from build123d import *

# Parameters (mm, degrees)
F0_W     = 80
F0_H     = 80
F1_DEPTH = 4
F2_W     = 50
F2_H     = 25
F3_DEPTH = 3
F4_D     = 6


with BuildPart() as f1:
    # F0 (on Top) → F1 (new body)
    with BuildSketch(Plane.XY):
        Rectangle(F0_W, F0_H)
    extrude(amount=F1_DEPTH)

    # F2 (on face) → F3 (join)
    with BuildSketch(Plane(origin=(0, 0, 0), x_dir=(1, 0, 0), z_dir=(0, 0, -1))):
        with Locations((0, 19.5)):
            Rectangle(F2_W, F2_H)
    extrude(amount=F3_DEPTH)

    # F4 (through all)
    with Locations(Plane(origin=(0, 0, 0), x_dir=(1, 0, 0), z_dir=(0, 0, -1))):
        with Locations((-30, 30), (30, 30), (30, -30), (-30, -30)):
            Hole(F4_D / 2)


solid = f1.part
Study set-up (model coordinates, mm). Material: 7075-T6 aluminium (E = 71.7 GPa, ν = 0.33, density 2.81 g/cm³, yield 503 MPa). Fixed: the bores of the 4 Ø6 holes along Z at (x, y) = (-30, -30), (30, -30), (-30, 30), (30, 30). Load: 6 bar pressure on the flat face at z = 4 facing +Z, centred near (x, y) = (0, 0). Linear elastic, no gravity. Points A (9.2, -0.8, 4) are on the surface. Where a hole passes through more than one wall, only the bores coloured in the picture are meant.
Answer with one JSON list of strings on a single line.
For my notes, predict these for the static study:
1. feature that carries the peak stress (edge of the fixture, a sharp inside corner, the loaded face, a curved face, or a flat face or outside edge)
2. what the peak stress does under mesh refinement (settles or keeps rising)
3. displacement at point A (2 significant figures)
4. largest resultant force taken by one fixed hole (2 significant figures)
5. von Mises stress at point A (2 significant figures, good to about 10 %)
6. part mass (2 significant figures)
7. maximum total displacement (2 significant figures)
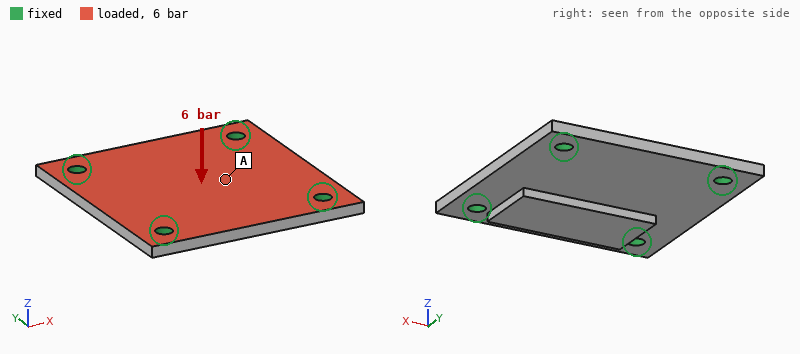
["edge of the fixture", "keeps rising", "84 µm", "1.1 kN", "32 MPa", "81 g", "92 µm"]
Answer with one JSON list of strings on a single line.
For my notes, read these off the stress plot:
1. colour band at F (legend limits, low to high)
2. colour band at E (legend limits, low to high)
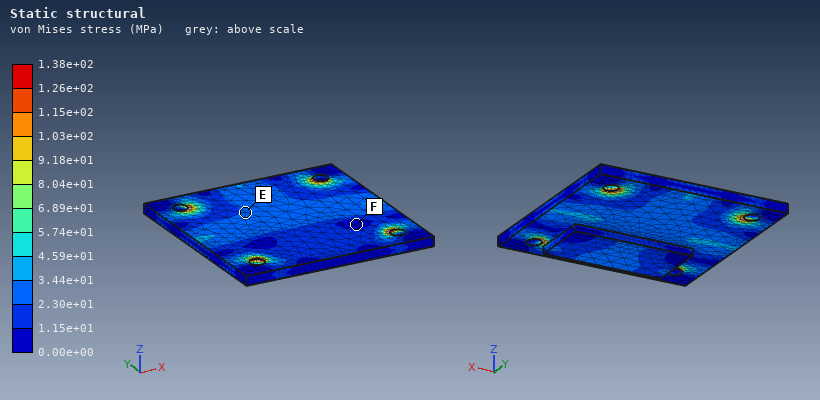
["0.00e+00 to 1.15e+01 MPa", "2.30e+01 to 3.44e+01 MPa"]
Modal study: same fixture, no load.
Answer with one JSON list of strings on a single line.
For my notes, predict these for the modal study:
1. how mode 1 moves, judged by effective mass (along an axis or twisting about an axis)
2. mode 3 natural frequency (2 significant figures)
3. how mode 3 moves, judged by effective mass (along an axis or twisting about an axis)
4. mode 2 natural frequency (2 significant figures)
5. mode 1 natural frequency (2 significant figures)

["along Z", "7200 Hz", "twisting about Y", "6800 Hz", "4400 Hz"]
